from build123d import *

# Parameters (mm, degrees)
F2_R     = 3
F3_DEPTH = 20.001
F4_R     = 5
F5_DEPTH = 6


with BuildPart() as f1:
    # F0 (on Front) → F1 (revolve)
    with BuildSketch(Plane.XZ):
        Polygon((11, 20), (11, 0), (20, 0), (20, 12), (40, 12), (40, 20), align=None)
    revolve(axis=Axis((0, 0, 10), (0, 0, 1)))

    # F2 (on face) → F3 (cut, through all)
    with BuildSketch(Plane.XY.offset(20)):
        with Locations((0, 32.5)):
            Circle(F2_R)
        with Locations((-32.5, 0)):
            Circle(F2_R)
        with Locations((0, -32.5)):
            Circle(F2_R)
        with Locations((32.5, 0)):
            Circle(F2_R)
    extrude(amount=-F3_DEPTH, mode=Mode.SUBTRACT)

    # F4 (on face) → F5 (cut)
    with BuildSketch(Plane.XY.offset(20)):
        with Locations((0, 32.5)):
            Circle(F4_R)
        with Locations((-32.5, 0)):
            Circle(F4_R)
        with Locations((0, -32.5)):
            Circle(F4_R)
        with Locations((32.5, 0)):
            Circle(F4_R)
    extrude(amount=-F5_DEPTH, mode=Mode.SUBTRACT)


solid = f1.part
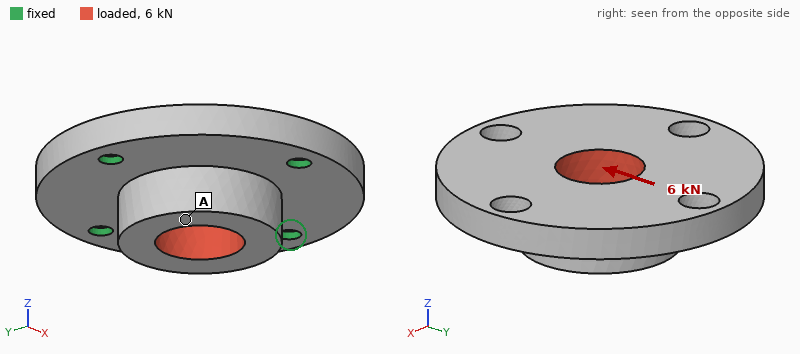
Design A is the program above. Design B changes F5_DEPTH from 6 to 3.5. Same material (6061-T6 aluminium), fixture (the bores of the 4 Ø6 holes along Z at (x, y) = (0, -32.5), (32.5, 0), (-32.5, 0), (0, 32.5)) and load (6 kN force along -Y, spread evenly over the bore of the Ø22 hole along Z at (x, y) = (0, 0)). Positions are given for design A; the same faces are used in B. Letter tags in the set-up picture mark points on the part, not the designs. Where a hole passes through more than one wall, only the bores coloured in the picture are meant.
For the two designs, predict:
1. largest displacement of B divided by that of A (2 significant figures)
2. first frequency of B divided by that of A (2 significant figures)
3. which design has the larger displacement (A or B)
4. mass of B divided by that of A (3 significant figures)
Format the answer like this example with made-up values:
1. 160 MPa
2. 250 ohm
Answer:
1. 0.76
2. 1.2
3. A
4. 1.01
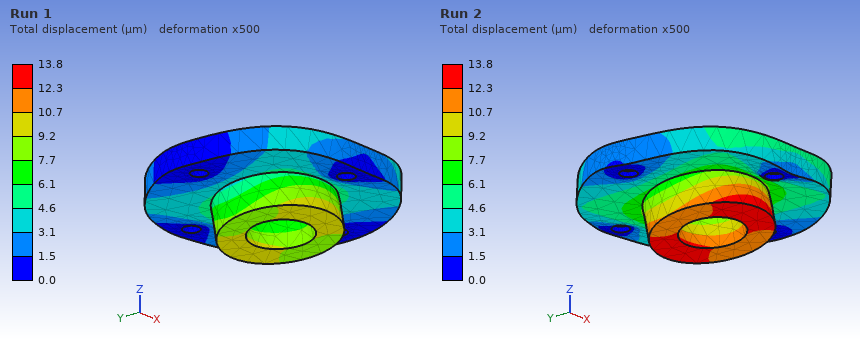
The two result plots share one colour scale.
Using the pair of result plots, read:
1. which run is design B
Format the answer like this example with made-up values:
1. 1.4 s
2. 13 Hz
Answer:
1. Run 1
